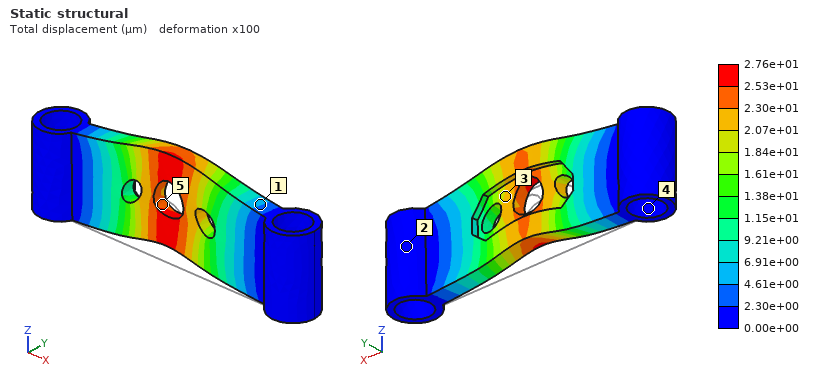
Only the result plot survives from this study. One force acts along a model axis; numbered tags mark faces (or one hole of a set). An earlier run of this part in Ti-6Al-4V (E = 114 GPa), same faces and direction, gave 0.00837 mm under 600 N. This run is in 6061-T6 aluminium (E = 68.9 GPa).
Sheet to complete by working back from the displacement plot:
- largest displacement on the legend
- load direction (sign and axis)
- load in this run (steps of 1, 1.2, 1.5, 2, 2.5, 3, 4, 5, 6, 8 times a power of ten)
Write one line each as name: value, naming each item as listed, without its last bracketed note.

largest displacement on the legend: 2.76e+01 µm
load direction: +Z
load in this run: 1.2 kN
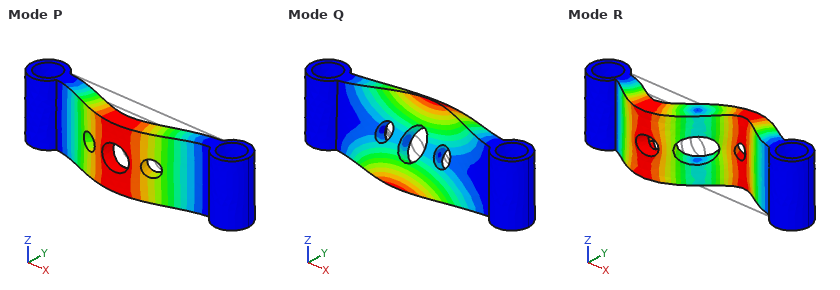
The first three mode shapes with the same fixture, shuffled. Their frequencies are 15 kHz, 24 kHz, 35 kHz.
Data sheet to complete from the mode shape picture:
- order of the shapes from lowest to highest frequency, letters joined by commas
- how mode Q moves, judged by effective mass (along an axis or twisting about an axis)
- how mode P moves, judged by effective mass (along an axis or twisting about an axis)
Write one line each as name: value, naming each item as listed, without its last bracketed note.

order of the shapes from lowest to highest frequency, letters joined by commas: P, Q, R
how mode Q moves, judged by effective mass: twisting about X
how mode P moves, judged by effective mass: along Y
